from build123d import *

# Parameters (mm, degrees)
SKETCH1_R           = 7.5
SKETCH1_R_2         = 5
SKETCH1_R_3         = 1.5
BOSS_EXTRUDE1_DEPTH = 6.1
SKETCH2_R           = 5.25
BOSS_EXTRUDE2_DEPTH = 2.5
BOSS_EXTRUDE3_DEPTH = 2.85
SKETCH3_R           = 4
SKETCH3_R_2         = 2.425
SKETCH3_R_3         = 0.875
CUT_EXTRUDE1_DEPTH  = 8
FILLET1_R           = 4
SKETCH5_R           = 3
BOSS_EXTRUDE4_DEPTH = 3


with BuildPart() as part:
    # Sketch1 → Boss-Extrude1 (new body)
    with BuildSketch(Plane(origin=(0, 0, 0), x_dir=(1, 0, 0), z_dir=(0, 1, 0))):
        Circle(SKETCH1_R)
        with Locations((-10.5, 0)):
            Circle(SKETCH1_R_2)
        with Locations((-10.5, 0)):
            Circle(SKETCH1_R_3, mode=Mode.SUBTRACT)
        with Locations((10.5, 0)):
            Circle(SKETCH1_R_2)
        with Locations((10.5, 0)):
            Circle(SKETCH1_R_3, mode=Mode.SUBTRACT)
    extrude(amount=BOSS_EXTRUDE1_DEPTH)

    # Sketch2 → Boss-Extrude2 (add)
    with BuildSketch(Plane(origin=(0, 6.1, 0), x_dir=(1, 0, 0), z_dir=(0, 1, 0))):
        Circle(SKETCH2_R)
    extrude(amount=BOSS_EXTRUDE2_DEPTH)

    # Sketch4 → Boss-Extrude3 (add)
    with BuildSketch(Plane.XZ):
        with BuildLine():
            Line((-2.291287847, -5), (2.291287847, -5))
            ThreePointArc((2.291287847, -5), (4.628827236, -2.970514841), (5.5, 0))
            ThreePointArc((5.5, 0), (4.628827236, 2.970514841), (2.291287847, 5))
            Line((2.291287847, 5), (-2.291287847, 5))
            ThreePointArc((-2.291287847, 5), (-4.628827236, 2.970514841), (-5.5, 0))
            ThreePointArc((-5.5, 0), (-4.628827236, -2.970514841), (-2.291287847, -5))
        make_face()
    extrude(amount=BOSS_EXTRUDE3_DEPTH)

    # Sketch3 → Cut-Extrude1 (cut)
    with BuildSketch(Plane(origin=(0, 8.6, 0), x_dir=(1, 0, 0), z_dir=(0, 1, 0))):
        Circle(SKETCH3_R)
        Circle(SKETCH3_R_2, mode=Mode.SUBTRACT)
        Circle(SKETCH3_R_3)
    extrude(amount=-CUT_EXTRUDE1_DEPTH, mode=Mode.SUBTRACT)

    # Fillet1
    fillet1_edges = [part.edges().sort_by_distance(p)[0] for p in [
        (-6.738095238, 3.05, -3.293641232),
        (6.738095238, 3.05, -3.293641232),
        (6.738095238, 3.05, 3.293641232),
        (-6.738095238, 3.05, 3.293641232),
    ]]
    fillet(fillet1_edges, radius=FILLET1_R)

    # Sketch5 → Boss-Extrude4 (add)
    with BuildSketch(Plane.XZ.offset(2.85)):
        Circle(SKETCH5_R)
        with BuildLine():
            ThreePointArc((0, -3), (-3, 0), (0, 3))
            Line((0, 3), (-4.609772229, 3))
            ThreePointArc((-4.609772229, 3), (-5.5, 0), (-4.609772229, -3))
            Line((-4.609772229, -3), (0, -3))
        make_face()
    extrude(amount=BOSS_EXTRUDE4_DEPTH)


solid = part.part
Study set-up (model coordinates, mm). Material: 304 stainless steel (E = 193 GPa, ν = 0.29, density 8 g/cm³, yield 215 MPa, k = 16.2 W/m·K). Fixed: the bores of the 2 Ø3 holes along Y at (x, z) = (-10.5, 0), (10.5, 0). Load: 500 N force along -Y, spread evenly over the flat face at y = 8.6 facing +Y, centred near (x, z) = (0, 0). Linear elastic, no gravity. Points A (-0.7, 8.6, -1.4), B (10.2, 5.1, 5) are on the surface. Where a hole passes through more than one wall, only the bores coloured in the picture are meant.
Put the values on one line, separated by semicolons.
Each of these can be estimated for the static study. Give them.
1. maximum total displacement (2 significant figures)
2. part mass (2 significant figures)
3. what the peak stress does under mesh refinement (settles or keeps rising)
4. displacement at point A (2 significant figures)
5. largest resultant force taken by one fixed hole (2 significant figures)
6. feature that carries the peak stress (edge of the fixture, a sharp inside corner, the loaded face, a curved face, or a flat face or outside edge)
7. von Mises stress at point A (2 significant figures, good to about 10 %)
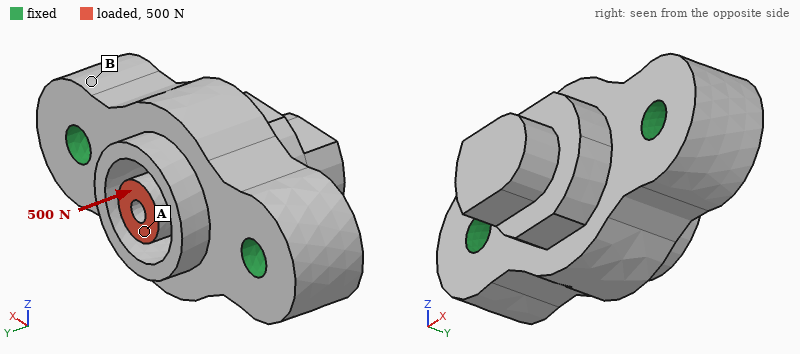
2.5 µm; 18 g; keeps rising; 2.4 µm; 270 N; edge of the fixture; 31 MPa
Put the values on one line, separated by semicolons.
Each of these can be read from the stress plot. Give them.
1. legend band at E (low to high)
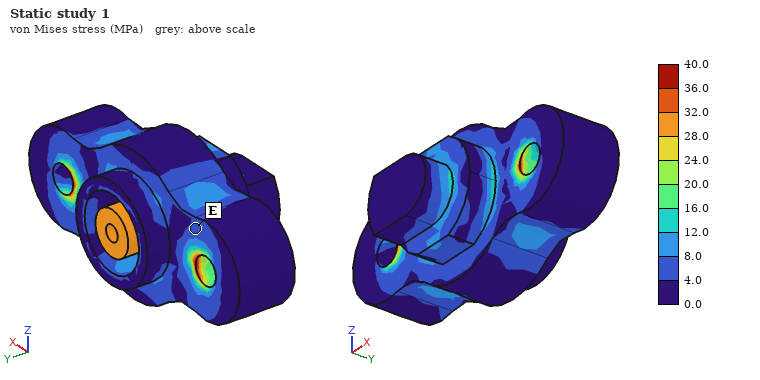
4.0 to 8.0 MPa
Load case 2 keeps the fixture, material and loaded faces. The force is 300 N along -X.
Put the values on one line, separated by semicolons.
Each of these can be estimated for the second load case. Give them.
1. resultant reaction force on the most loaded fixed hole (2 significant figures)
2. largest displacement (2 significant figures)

200 N; 20 µm
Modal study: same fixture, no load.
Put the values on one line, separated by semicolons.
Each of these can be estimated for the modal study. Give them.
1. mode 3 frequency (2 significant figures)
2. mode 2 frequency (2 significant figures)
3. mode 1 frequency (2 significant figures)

34 kHz; 34 kHz; 29 kHz
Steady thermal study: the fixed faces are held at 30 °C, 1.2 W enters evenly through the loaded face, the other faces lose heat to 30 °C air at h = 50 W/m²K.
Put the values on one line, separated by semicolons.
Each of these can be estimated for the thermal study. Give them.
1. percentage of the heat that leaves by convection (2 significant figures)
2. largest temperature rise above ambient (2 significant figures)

32 %; 42 K
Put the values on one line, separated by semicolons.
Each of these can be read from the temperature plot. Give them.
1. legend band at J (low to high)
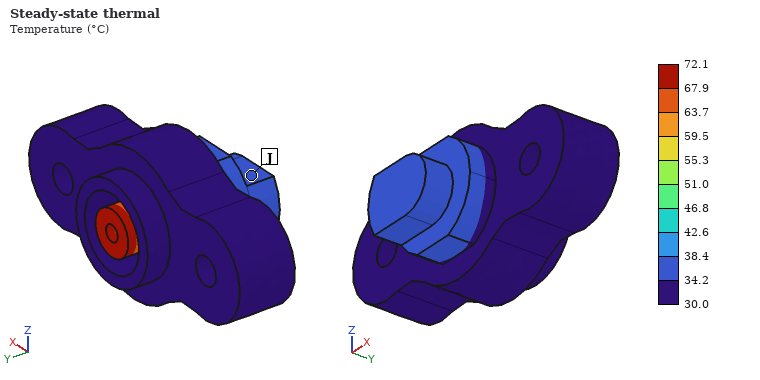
34.2 to 38.4 °C
